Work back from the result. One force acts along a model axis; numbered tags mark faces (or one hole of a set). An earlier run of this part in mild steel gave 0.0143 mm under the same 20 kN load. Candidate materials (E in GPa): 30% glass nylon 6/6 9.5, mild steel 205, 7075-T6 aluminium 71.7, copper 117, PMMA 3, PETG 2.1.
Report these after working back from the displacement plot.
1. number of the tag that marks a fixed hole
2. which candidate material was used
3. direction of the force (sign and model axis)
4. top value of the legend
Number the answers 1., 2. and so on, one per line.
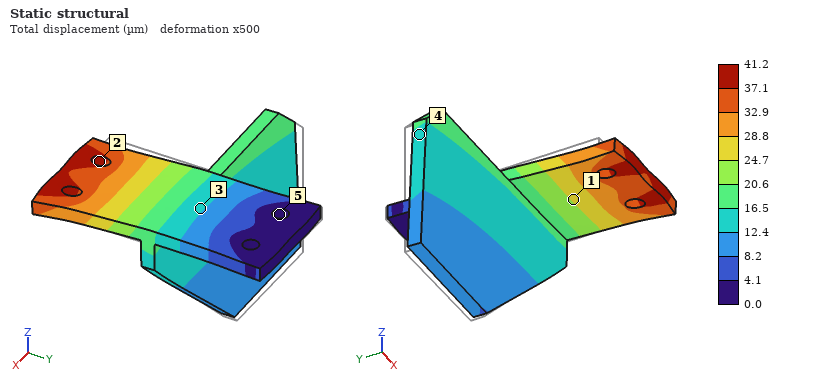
1. 5
2. 7075-T6 aluminium
3. -Y
4. 41.2 µm
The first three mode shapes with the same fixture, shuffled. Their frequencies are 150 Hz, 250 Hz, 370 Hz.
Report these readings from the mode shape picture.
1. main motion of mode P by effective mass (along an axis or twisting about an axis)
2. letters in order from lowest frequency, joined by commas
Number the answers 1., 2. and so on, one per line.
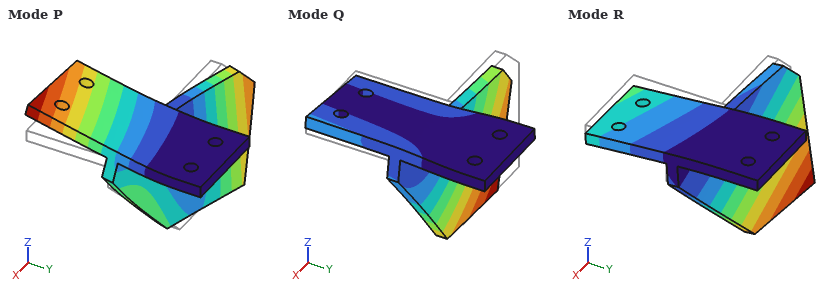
1. along Z
2. R, Q, P
